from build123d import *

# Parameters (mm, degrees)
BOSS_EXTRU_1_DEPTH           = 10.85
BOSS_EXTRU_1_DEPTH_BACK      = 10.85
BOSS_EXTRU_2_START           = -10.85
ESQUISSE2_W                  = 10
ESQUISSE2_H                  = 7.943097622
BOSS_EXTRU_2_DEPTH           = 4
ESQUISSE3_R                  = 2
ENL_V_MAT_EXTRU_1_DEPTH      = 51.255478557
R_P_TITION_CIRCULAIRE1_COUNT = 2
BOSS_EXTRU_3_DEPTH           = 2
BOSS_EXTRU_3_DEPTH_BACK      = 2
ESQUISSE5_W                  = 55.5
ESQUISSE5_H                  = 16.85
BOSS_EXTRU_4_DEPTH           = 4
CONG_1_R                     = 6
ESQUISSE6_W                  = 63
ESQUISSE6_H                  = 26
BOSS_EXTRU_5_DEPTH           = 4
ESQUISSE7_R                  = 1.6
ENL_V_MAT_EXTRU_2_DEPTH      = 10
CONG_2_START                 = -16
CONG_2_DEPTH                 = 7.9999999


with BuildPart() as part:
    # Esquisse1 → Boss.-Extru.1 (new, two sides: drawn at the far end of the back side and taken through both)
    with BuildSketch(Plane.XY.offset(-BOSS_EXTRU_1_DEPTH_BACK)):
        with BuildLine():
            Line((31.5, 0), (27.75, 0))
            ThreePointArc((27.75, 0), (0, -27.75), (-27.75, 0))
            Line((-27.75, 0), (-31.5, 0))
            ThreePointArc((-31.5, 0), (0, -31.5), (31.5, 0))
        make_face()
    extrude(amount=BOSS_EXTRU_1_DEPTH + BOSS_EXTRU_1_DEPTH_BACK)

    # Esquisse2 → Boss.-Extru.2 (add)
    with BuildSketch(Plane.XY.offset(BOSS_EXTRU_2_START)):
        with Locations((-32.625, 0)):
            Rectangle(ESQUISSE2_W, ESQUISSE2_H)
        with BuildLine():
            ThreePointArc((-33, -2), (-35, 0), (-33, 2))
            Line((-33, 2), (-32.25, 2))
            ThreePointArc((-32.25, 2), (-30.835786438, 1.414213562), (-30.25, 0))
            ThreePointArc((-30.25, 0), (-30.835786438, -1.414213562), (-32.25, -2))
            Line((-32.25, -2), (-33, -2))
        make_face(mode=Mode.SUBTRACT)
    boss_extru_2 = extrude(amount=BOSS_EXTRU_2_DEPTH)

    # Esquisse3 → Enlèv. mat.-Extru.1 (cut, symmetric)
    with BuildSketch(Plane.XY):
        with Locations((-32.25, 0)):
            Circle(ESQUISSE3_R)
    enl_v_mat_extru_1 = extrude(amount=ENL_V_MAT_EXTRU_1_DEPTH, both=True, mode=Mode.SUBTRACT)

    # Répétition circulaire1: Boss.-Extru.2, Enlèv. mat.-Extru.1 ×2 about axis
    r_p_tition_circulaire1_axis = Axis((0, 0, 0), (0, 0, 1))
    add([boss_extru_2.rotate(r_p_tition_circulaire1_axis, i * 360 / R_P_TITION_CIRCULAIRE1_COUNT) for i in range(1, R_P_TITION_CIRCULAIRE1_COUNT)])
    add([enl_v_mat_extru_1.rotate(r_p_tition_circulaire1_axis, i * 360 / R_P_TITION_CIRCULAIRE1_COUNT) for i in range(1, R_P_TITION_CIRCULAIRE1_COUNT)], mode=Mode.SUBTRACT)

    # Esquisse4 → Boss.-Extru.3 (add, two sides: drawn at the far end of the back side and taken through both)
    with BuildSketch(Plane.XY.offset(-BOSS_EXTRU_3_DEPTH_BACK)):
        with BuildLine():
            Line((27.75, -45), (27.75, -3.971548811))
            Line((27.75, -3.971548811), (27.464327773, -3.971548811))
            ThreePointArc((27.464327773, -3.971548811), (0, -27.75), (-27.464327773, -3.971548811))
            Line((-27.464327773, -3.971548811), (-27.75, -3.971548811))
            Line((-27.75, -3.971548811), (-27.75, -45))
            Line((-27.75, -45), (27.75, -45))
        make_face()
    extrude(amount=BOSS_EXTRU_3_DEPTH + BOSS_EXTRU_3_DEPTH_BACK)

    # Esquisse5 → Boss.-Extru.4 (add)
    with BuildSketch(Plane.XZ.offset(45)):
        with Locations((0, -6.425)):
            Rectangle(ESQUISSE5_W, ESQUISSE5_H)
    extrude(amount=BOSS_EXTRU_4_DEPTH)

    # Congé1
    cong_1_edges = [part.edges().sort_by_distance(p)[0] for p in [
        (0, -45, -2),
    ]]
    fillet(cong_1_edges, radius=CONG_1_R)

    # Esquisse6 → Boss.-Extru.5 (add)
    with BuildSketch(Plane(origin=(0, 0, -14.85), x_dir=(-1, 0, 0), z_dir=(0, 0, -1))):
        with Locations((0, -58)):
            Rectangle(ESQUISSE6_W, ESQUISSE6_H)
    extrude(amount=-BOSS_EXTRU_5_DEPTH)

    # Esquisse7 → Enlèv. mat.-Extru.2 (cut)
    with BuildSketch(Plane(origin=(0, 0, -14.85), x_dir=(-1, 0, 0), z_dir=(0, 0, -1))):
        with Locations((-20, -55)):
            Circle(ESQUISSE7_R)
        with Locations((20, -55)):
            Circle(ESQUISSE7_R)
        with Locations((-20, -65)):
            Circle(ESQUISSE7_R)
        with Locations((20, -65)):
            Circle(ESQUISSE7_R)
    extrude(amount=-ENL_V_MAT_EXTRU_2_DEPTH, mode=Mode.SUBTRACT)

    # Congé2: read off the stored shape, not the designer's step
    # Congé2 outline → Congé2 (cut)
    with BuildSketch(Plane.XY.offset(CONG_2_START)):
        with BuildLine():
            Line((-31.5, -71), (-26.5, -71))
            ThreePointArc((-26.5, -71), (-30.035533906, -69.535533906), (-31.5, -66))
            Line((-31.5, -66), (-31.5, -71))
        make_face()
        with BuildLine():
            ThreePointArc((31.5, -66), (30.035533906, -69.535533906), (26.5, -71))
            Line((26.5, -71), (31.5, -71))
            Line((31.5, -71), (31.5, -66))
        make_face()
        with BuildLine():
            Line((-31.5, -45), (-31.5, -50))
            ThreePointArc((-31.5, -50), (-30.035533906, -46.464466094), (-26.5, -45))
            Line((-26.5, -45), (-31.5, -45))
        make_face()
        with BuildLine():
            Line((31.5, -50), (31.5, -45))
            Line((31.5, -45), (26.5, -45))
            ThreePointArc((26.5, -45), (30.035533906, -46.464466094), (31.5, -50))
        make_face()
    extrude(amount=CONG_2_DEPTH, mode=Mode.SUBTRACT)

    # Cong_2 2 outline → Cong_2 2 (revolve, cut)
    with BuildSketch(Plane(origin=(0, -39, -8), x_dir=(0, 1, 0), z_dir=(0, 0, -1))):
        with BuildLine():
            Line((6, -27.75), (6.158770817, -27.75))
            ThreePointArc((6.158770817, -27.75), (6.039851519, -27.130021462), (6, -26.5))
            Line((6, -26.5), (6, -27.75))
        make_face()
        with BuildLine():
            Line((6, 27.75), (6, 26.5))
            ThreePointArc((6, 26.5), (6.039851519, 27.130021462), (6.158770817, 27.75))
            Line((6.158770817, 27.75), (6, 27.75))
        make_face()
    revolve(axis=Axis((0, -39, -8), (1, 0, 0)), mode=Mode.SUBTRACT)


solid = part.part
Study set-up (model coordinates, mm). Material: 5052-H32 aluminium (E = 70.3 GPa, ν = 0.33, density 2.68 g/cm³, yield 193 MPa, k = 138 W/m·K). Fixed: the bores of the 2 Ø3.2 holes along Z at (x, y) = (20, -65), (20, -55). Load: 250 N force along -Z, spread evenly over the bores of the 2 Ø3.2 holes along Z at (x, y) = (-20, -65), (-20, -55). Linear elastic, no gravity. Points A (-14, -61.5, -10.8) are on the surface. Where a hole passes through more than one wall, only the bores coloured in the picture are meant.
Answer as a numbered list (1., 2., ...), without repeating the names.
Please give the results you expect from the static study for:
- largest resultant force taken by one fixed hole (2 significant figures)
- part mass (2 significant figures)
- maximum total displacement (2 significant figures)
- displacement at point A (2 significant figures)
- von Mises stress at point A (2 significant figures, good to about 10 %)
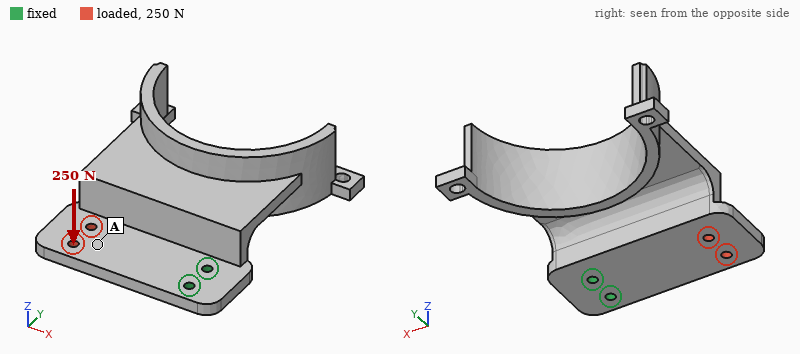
1. 130 N
2. 58 g
3. 0.29 mm
4. 0.17 mm
5. 18 MPa
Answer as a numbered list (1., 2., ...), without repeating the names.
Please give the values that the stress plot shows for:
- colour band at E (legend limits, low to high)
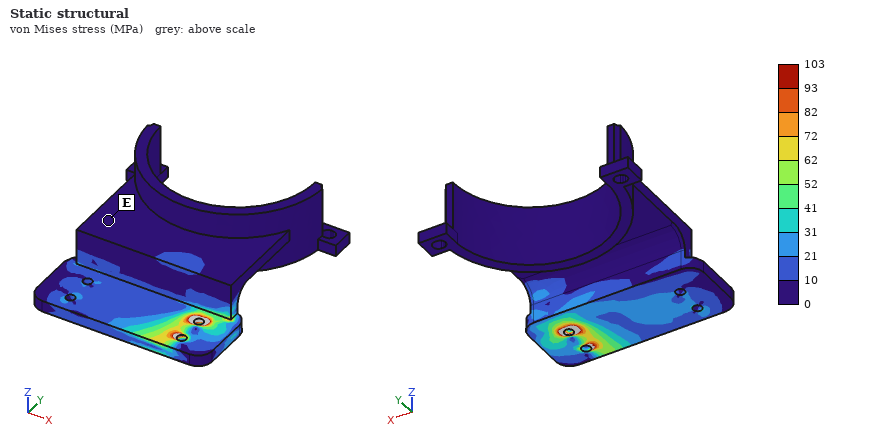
1. 0 to 10 MPa
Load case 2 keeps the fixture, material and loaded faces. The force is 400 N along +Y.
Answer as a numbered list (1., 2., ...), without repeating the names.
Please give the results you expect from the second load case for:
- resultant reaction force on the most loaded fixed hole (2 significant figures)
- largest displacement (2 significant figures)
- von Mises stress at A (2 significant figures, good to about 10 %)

1. 1.3 kN
2. 78 µm
3. 9.0 MPa
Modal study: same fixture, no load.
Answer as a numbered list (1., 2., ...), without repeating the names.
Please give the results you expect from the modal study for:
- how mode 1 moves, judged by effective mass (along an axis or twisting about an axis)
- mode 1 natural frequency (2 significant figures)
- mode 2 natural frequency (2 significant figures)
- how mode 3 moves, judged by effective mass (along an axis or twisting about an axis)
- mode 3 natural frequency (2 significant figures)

1. along Z
2. 650 Hz
3. 1200 Hz
4. along X
5. 1700 Hz
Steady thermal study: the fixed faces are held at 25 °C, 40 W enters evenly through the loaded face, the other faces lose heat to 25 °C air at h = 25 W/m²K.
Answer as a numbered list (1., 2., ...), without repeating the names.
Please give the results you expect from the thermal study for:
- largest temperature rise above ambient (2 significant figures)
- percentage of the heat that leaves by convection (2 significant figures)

1. 79 K
2. 23 %
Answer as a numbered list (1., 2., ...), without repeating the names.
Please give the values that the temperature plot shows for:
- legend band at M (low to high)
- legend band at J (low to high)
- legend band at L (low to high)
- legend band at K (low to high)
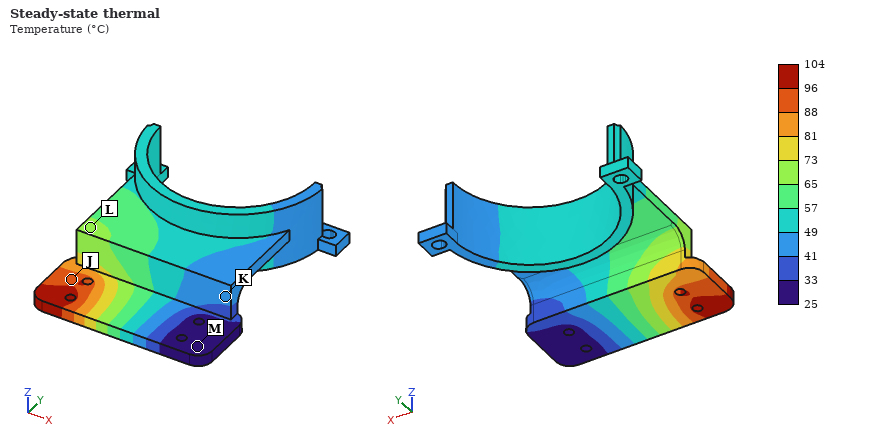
1. 25 to 33 °C
2. 88 to 96 °C
3. 65 to 73 °C
4. 41 to 49 °C
